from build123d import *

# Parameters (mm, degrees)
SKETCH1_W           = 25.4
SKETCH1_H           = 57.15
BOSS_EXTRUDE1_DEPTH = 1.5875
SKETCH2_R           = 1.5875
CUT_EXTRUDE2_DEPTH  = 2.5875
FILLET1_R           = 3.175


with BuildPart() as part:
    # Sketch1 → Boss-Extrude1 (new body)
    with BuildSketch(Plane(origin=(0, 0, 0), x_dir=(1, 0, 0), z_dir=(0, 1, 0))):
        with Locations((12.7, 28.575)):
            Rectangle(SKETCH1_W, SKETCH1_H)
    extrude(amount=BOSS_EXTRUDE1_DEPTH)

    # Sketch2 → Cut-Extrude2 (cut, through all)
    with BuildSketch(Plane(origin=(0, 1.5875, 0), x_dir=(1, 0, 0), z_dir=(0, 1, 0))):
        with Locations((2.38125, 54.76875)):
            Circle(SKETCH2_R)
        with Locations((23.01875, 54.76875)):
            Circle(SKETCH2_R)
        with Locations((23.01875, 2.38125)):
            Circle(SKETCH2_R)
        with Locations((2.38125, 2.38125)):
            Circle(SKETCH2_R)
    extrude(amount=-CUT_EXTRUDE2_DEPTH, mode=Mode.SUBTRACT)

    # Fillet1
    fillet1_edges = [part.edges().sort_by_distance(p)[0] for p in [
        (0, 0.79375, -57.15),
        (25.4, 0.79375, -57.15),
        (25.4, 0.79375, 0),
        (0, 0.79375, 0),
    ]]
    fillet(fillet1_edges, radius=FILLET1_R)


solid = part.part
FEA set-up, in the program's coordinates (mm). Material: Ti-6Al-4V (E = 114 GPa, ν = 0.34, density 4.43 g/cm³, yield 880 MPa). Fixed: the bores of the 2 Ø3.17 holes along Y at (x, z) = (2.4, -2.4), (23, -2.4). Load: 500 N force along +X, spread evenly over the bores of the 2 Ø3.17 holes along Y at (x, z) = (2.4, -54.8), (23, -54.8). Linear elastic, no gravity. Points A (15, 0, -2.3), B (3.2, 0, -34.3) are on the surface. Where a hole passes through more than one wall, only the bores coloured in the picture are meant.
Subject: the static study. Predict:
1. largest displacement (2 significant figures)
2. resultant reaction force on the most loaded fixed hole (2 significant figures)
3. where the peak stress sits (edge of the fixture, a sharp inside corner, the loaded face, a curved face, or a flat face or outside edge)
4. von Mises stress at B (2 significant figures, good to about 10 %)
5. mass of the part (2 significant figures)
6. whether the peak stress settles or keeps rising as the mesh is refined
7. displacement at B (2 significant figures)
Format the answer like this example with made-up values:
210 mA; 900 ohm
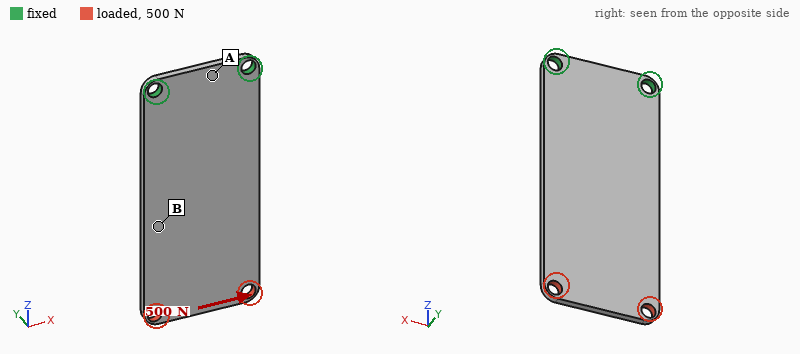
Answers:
0.12 mm; 1.3 kN; edge of the fixture; 47 MPa; 9.9 g; keeps rising; 0.057 mm
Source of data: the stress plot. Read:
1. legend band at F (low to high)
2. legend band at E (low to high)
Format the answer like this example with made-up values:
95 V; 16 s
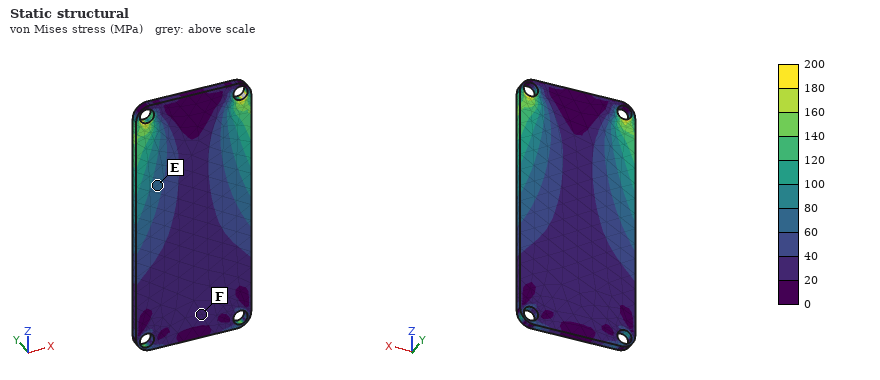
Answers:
20 to 40 MPa; 60 to 80 MPa
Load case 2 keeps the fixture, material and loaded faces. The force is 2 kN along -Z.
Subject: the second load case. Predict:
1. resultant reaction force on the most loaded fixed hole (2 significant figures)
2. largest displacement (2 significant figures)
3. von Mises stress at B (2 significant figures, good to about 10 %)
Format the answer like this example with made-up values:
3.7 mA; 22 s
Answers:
1.0 kN; 45 µm; 51 MPa
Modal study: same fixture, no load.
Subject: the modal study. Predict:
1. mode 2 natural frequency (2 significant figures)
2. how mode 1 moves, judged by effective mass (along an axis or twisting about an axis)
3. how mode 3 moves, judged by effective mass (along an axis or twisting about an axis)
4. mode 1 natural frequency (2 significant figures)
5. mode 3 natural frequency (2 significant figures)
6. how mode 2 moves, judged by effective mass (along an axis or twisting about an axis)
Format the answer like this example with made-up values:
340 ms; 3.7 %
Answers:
2100 Hz; along Y; along Y; 440 Hz; 2800 Hz; twisting about Z
